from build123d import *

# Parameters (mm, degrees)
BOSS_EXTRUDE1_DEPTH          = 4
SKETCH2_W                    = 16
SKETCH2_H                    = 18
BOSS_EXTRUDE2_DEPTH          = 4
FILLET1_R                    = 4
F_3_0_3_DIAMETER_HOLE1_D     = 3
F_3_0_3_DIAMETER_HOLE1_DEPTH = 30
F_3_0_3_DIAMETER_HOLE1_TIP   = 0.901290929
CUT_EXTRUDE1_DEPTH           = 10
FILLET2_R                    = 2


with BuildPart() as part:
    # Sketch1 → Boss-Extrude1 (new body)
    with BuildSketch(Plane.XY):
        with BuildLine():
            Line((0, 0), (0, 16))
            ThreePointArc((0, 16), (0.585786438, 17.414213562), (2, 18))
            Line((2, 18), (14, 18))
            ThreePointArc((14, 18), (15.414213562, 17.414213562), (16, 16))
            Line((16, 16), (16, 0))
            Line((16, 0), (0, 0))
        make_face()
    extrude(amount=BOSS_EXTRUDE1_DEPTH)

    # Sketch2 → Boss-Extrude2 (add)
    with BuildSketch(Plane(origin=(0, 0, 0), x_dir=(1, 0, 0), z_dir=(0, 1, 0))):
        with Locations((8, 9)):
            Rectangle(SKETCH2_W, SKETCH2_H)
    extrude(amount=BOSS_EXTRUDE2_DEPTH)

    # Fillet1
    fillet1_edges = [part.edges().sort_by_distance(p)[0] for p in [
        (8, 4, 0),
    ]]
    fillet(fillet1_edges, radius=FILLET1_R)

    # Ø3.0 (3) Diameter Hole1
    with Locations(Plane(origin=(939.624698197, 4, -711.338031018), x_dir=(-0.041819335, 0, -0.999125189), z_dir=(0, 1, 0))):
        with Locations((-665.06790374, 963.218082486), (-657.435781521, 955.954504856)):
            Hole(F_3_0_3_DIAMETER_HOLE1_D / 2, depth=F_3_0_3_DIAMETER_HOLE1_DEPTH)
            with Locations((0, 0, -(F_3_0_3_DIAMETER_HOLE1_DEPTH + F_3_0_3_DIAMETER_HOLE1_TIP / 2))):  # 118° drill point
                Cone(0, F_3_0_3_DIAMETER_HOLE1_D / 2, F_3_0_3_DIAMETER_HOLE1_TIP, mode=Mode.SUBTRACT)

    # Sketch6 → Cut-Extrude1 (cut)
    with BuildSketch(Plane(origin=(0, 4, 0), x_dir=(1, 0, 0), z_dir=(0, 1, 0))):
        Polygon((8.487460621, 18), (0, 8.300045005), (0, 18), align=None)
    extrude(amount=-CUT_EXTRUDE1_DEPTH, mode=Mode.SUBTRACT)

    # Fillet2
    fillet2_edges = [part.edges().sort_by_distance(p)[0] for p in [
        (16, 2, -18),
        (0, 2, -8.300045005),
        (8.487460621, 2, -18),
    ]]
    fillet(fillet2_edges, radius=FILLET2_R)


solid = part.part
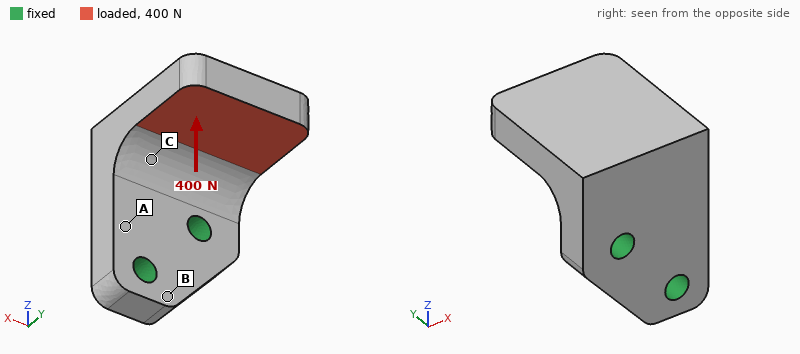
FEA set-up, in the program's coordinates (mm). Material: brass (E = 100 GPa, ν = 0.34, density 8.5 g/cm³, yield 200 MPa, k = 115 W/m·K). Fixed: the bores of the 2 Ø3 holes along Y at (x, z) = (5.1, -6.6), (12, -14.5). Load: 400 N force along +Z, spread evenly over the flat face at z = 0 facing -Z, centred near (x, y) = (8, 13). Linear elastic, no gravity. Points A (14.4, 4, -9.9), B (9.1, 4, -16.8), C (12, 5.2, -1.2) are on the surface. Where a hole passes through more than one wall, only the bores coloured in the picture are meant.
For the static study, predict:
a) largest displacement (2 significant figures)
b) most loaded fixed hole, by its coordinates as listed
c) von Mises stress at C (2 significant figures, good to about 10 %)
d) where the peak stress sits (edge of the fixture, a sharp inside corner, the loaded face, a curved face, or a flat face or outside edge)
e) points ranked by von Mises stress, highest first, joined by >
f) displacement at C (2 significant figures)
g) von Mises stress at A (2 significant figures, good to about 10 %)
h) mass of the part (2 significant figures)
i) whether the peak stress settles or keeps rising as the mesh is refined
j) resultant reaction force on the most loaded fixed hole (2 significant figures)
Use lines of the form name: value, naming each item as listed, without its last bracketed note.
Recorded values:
largest displacement: 76 µm
most loaded fixed hole, by its coordinates as listed: (5.1, -6.6)
von Mises stress at C: 75 MPa
where the peak stress sits: edge of the fixture
points ranked by von Mises stress, highest first, joined by >: C > A > B
displacement at C: 14 µm
von Mises stress at A: 34 MPa
mass of the part: 18 g
whether the peak stress settles or keeps rising as the mesh is refined: keeps rising
resultant reaction force on the most loaded fixed hole: 310 N
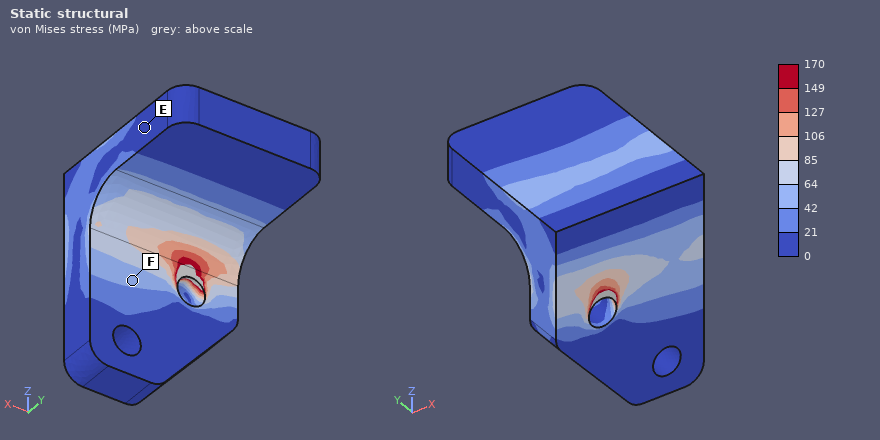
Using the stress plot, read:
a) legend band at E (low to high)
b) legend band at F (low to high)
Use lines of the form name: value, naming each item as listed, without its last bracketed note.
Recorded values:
legend band at E: 0 to 21 MPa
legend band at F: 42 to 64 MPa
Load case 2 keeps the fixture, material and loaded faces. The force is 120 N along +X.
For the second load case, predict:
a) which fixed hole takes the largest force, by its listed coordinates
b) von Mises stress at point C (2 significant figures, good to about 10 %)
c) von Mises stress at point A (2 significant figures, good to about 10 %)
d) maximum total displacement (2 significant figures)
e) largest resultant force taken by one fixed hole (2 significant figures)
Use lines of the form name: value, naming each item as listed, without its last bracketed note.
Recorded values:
which fixed hole takes the largest force, by its listed coordinates: (5.1, -6.6)
von Mises stress at point C: 18 MPa
von Mises stress at point A: 11 MPa
maximum total displacement: 14 µm
largest resultant force taken by one fixed hole: 150 N
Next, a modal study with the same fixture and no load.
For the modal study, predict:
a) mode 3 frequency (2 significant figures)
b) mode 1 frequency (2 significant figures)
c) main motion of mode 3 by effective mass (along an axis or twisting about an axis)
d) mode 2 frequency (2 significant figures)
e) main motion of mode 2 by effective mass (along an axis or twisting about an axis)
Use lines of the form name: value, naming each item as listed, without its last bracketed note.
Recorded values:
mode 3 frequency: 16 kHz
mode 1 frequency: 5100 Hz
main motion of mode 3 by effective mass: along Y
mode 2 frequency: 7200 Hz
main motion of mode 2 by effective mass: along X
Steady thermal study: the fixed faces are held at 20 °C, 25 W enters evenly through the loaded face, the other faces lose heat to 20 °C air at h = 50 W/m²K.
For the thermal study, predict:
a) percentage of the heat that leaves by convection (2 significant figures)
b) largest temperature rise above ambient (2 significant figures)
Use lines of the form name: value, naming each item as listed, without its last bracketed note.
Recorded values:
percentage of the heat that leaves by convection: 5.6 %
largest temperature rise above ambient: 57 K
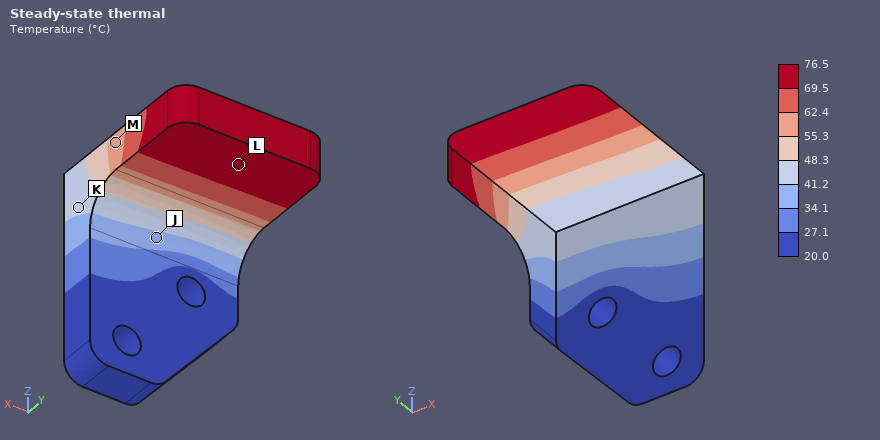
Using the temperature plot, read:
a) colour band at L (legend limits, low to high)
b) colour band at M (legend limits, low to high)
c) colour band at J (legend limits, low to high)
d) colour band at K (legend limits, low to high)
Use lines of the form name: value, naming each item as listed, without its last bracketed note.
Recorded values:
colour band at L: 69.5 to 76.5 °C
colour band at M: 55.3 to 62.4 °C
colour band at J: 34.1 to 41.2 °C
colour band at K: 41.2 to 48.3 °C
